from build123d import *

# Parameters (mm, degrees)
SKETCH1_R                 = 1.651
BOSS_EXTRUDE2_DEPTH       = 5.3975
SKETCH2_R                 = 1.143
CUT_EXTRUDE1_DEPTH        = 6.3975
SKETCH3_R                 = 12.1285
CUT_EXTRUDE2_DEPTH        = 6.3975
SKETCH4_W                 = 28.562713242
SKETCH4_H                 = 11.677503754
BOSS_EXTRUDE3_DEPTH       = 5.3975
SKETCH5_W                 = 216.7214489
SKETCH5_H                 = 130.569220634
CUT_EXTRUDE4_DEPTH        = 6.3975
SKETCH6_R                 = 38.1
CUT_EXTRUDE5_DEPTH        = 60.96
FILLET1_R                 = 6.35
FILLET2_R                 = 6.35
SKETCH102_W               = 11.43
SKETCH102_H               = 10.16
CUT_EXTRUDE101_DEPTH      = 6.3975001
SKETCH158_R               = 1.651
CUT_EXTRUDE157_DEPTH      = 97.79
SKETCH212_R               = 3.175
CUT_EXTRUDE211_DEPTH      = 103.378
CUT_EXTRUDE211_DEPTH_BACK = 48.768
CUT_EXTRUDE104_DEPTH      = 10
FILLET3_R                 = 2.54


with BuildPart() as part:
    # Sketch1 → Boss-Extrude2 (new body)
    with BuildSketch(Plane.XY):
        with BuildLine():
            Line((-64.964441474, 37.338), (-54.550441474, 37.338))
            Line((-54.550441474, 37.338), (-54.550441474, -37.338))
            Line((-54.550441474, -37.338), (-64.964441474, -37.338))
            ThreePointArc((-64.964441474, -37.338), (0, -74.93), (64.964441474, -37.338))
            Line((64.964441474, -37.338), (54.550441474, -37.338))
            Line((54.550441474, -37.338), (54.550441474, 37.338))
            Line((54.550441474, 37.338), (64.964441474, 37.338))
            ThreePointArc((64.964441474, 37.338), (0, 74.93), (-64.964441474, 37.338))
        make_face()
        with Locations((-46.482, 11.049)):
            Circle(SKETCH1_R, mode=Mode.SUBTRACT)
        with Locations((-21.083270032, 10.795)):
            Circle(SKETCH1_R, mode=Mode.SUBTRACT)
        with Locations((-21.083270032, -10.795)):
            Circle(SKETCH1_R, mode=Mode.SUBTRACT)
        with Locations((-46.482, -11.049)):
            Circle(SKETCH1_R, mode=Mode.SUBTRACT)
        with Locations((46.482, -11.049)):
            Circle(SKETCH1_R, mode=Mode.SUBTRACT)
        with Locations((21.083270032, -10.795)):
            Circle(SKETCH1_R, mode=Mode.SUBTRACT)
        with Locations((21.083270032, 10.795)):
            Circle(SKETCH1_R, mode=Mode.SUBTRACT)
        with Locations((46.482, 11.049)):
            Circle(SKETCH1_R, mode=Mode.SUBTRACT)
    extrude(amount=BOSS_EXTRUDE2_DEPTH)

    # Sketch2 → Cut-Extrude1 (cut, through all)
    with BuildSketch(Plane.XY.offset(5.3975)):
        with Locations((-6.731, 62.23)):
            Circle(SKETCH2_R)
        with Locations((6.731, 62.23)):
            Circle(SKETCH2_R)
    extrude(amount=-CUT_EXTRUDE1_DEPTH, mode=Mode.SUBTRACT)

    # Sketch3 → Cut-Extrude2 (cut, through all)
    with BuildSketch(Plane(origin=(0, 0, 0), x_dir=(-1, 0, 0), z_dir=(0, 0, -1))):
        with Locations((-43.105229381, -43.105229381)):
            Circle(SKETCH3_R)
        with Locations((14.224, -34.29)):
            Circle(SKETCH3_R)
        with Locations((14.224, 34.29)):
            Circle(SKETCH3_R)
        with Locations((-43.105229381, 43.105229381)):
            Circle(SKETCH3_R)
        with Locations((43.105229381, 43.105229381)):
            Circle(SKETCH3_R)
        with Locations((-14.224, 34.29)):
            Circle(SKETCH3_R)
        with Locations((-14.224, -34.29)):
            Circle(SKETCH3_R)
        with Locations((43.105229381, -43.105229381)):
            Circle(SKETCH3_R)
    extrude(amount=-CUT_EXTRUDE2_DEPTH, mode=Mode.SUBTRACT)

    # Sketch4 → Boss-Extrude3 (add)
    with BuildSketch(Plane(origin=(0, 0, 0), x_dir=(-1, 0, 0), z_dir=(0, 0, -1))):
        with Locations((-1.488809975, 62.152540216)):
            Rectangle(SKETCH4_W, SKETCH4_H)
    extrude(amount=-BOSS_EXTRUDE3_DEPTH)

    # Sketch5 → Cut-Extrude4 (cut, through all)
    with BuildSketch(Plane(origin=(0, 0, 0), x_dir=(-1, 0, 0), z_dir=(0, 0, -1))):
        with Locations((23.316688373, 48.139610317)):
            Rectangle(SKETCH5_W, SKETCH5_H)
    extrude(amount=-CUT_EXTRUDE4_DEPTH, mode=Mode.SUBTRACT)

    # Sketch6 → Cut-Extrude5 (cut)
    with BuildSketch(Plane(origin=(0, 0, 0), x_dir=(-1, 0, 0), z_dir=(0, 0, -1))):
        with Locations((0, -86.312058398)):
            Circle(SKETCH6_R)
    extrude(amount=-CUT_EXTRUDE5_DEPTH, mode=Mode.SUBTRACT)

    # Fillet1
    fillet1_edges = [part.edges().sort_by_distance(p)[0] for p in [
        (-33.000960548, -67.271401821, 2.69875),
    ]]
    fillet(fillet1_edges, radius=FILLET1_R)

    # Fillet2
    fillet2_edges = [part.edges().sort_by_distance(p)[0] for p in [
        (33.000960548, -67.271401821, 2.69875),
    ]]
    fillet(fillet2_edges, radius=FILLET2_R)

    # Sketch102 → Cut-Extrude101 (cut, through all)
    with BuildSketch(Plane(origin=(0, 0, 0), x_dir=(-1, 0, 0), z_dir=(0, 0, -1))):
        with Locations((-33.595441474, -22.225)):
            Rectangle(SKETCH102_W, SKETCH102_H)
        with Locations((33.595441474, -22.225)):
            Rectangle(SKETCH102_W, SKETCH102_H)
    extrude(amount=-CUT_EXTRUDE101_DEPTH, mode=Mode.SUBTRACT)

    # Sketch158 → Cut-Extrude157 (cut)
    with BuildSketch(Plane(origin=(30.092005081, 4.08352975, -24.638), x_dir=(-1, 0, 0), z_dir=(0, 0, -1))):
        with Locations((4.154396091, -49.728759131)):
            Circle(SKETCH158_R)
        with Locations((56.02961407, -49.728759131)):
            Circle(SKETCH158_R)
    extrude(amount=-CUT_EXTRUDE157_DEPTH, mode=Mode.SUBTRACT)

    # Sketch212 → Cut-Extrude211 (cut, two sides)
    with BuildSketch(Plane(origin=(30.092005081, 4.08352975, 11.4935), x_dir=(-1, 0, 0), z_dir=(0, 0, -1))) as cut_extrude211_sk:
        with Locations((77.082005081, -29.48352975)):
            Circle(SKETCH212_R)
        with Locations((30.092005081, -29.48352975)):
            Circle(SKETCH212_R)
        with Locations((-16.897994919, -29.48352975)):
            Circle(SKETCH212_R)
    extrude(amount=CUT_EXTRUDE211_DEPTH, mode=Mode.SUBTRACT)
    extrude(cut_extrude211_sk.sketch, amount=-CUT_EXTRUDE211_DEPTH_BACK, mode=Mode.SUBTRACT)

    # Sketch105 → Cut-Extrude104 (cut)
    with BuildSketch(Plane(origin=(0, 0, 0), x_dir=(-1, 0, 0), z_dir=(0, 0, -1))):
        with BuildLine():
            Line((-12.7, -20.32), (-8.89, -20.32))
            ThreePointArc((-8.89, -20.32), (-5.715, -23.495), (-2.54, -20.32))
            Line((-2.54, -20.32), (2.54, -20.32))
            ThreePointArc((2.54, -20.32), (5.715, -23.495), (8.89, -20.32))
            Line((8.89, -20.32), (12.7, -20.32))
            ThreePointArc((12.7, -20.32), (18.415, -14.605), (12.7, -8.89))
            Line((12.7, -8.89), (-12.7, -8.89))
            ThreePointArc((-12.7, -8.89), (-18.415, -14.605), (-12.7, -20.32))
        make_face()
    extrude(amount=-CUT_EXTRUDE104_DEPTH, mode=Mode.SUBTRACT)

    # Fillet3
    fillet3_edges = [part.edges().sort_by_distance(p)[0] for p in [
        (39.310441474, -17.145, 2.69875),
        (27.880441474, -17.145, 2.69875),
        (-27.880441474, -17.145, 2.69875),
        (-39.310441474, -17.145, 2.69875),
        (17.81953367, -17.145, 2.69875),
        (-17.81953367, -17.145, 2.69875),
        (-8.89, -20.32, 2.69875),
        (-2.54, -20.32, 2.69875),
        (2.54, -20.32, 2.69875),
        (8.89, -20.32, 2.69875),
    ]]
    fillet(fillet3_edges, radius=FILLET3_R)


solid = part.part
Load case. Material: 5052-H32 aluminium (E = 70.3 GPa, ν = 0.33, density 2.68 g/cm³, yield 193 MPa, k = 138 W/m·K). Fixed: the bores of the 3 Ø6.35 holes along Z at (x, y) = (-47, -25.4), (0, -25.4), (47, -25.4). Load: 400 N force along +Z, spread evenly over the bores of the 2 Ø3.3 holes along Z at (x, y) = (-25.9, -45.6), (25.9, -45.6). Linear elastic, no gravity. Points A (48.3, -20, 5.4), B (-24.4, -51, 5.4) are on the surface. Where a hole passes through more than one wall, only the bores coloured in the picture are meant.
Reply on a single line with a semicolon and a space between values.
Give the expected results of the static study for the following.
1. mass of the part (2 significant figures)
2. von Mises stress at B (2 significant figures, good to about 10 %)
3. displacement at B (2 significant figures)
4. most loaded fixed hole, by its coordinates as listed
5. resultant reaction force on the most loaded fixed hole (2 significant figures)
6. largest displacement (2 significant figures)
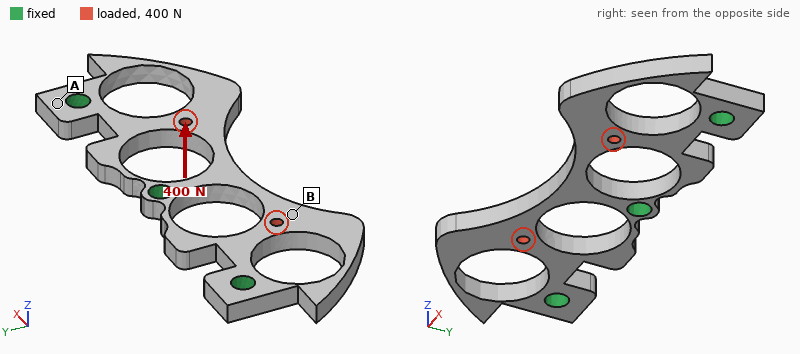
30 g; 19 MPa; 0.11 mm; (0, -25.4); 160 N; 0.17 mm
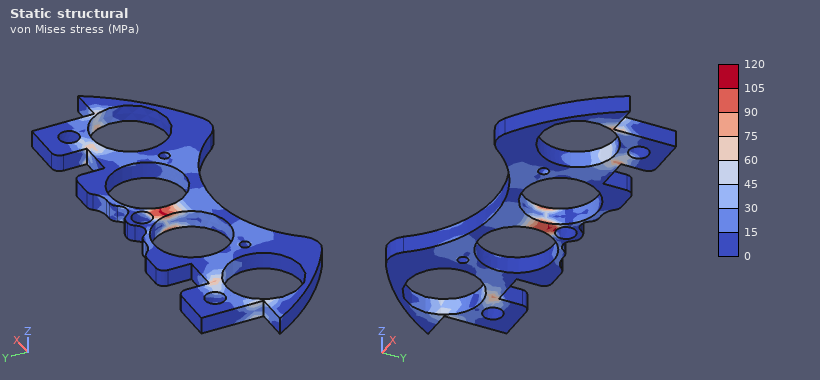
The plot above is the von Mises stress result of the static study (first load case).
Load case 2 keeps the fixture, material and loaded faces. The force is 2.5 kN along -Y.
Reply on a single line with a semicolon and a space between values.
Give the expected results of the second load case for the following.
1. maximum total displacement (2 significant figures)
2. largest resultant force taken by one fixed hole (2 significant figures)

44 µm; 1.1 kN
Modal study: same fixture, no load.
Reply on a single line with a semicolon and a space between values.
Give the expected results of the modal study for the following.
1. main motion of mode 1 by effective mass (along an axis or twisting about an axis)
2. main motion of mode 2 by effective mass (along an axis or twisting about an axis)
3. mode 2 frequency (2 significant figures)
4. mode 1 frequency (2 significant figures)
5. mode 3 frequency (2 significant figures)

along Z; twisting about Y; 2300 Hz; 2100 Hz; 5900 Hz
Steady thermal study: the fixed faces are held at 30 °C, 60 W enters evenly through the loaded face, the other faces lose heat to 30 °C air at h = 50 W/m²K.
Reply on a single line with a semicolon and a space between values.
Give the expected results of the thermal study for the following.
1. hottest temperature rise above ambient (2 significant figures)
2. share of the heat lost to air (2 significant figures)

82 K; 24 %
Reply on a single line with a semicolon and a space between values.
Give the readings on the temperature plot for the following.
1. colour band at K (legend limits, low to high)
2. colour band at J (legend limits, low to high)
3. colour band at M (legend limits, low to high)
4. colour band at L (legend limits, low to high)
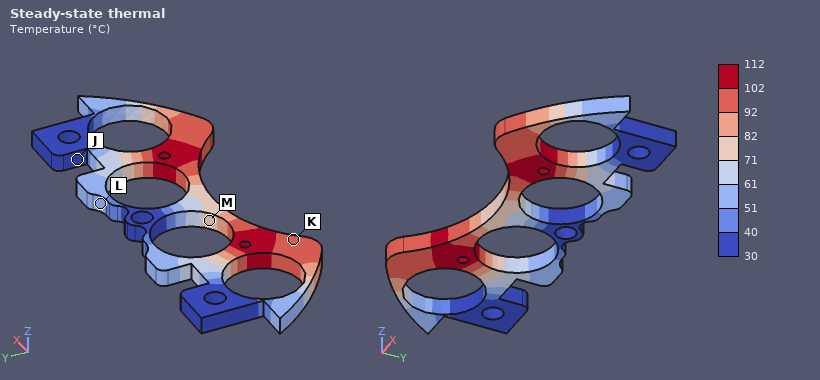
92 to 102 °C; 30 to 40 °C; 71 to 82 °C; 51 to 61 °C
